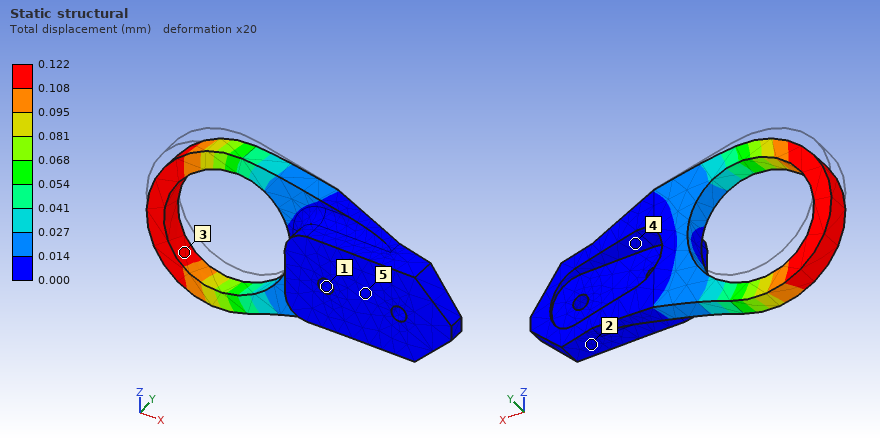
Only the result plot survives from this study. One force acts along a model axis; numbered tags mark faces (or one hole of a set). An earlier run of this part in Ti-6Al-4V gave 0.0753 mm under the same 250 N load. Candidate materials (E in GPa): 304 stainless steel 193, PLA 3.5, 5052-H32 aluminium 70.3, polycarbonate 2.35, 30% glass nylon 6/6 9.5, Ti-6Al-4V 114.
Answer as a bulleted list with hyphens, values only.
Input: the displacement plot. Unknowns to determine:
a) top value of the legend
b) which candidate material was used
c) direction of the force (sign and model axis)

- 0.122 mm
- 5052-H32 aluminium
- -Z
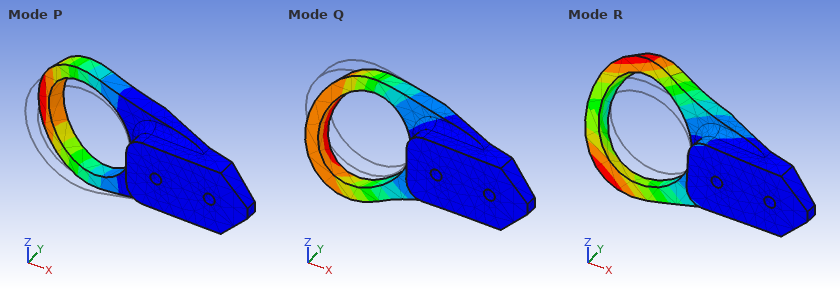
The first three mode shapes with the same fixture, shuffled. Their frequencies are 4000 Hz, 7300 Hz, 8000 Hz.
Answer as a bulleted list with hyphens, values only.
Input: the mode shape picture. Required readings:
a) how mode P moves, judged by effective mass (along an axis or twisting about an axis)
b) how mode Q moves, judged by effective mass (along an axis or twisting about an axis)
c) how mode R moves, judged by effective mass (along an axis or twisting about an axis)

- along Y
- along Z
- twisting about X
